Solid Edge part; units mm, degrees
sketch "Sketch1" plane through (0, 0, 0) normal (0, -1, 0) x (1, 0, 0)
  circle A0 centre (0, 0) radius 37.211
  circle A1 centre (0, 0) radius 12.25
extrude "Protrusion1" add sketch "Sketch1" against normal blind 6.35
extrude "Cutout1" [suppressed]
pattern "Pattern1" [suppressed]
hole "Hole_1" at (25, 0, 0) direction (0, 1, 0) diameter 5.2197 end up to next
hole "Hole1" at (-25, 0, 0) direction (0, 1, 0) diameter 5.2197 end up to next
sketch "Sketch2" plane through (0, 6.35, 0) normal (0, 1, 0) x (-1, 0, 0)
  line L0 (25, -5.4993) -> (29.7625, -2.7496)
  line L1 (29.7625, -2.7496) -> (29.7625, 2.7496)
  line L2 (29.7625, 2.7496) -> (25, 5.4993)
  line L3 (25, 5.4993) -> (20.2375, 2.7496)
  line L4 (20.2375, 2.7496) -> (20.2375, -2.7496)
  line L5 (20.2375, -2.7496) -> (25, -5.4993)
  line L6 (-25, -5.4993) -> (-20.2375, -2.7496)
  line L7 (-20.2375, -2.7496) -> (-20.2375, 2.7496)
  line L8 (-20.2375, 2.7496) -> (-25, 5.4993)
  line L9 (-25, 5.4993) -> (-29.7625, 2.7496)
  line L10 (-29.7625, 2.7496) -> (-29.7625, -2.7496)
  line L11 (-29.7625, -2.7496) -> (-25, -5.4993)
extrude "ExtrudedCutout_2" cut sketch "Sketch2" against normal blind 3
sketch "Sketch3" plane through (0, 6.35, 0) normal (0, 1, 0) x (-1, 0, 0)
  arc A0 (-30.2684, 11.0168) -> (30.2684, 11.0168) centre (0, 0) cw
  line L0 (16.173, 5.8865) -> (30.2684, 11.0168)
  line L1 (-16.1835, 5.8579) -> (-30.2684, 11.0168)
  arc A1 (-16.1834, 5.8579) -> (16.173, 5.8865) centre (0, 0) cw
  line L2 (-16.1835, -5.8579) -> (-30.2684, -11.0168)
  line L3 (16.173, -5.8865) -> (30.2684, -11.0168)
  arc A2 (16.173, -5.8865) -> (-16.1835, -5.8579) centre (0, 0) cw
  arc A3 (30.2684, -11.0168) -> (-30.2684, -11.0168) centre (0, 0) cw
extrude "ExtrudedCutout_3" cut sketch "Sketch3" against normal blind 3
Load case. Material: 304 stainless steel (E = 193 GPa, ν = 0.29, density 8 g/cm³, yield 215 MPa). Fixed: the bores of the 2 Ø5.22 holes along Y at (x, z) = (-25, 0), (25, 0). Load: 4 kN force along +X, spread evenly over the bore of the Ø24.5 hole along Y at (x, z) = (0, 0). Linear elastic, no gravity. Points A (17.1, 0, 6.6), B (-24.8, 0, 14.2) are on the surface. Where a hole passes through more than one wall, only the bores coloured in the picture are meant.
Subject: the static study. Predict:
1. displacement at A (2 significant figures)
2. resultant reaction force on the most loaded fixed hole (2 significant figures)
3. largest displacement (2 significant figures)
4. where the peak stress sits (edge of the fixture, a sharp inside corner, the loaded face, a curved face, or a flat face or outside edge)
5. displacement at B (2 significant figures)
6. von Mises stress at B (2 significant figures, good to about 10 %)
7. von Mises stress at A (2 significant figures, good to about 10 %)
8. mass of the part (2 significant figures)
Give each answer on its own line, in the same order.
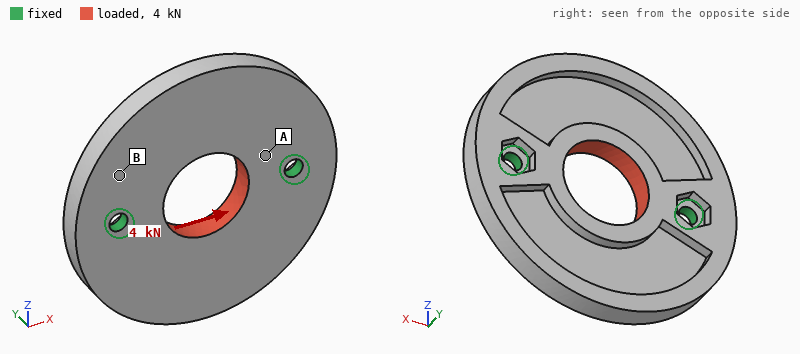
1.3 µm
2.0 kN
3.1 µm
edge of the fixture
1.7 µm
7.2 MPa
21 MPa
150 g
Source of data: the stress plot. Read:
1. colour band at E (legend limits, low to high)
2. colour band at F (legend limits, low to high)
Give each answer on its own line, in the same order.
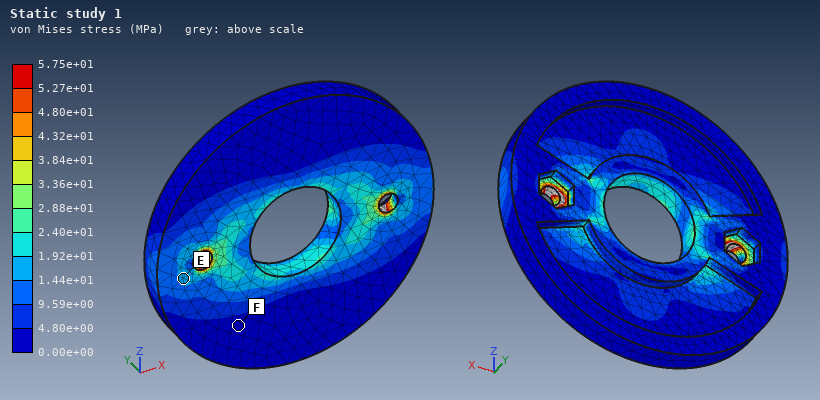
1.44e+01 to 1.92e+01 MPa
0.00e+00 to 4.80e+00 MPa
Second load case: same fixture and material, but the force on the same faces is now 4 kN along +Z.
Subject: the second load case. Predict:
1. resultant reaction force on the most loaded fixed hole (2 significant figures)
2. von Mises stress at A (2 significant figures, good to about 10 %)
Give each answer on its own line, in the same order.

2.0 kN
18 MPa
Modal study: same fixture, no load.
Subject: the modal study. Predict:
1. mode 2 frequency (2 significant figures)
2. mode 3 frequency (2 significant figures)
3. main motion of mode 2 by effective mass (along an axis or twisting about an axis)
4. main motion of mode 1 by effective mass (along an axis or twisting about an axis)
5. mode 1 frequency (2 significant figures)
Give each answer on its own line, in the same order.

3200 Hz
5700 Hz
along Y
twisting about X
2300 Hz
